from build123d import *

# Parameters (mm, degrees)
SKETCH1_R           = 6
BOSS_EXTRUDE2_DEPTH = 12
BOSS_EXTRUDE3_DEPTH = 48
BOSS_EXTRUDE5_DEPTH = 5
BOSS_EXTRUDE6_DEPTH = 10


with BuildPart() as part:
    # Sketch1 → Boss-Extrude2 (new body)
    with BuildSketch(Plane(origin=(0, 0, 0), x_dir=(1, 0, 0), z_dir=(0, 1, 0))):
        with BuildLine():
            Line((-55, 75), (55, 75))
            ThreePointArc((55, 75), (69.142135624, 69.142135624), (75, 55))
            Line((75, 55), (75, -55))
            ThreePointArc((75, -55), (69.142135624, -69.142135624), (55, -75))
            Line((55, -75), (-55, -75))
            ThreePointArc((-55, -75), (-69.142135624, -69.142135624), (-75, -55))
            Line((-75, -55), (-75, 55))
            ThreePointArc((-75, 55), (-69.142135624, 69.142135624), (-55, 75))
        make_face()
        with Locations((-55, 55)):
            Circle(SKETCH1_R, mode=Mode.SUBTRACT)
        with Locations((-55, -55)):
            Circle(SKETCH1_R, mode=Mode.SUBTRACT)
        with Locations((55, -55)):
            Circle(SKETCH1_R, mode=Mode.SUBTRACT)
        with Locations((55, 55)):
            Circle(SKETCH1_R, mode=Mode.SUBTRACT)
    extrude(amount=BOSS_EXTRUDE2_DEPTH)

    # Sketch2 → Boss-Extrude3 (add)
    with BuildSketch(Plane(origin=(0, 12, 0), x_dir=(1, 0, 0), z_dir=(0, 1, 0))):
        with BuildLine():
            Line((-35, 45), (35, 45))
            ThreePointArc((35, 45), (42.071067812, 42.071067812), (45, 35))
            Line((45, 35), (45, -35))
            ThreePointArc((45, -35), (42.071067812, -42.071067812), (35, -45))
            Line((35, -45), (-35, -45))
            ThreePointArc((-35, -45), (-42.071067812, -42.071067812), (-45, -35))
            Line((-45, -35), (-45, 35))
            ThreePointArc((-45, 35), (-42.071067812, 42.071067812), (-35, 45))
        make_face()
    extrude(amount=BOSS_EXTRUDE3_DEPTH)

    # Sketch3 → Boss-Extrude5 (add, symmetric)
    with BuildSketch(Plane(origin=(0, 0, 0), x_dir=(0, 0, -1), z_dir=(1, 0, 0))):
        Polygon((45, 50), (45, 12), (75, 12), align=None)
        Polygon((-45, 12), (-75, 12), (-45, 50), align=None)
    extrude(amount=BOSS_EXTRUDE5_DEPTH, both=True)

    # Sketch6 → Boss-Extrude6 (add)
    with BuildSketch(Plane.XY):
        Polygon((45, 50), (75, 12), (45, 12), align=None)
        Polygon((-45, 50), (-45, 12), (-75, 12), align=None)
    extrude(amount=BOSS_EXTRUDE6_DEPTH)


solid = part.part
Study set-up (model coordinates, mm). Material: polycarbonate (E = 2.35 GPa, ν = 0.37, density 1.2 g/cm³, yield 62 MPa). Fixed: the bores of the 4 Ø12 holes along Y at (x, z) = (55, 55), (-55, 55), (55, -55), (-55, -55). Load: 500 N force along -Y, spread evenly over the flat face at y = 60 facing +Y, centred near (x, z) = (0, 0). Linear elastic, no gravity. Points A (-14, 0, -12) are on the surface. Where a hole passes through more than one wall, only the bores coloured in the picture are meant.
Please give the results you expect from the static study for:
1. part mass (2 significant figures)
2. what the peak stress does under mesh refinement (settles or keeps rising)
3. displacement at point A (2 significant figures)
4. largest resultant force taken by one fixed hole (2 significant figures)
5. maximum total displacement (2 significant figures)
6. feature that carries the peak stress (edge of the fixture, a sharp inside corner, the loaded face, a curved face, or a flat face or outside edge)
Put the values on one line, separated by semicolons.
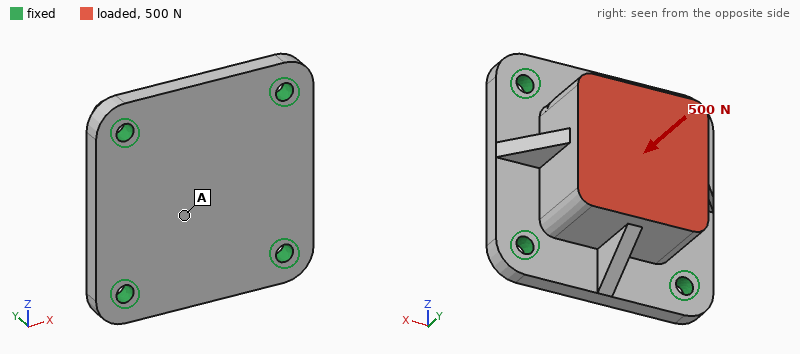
800 g; keeps rising; 21 µm; 130 N; 22 µm; edge of the fixture
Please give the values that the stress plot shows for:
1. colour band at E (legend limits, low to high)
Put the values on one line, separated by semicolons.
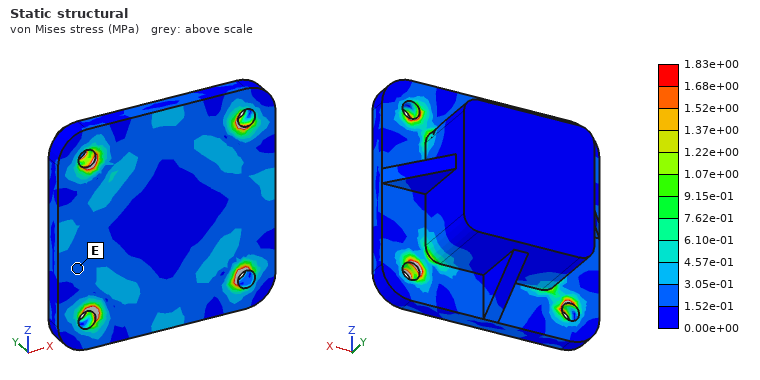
1.52e-01 to 3.05e-01 MPa
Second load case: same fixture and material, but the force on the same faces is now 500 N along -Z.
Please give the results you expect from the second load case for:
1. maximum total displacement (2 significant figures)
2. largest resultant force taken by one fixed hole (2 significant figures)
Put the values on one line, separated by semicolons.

40 µm; 200 N
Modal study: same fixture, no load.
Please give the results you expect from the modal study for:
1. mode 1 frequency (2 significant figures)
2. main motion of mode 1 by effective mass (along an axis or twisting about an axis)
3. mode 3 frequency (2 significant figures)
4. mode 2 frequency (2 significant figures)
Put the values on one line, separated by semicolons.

940 Hz; along Y; 1100 Hz; 1100 Hz
